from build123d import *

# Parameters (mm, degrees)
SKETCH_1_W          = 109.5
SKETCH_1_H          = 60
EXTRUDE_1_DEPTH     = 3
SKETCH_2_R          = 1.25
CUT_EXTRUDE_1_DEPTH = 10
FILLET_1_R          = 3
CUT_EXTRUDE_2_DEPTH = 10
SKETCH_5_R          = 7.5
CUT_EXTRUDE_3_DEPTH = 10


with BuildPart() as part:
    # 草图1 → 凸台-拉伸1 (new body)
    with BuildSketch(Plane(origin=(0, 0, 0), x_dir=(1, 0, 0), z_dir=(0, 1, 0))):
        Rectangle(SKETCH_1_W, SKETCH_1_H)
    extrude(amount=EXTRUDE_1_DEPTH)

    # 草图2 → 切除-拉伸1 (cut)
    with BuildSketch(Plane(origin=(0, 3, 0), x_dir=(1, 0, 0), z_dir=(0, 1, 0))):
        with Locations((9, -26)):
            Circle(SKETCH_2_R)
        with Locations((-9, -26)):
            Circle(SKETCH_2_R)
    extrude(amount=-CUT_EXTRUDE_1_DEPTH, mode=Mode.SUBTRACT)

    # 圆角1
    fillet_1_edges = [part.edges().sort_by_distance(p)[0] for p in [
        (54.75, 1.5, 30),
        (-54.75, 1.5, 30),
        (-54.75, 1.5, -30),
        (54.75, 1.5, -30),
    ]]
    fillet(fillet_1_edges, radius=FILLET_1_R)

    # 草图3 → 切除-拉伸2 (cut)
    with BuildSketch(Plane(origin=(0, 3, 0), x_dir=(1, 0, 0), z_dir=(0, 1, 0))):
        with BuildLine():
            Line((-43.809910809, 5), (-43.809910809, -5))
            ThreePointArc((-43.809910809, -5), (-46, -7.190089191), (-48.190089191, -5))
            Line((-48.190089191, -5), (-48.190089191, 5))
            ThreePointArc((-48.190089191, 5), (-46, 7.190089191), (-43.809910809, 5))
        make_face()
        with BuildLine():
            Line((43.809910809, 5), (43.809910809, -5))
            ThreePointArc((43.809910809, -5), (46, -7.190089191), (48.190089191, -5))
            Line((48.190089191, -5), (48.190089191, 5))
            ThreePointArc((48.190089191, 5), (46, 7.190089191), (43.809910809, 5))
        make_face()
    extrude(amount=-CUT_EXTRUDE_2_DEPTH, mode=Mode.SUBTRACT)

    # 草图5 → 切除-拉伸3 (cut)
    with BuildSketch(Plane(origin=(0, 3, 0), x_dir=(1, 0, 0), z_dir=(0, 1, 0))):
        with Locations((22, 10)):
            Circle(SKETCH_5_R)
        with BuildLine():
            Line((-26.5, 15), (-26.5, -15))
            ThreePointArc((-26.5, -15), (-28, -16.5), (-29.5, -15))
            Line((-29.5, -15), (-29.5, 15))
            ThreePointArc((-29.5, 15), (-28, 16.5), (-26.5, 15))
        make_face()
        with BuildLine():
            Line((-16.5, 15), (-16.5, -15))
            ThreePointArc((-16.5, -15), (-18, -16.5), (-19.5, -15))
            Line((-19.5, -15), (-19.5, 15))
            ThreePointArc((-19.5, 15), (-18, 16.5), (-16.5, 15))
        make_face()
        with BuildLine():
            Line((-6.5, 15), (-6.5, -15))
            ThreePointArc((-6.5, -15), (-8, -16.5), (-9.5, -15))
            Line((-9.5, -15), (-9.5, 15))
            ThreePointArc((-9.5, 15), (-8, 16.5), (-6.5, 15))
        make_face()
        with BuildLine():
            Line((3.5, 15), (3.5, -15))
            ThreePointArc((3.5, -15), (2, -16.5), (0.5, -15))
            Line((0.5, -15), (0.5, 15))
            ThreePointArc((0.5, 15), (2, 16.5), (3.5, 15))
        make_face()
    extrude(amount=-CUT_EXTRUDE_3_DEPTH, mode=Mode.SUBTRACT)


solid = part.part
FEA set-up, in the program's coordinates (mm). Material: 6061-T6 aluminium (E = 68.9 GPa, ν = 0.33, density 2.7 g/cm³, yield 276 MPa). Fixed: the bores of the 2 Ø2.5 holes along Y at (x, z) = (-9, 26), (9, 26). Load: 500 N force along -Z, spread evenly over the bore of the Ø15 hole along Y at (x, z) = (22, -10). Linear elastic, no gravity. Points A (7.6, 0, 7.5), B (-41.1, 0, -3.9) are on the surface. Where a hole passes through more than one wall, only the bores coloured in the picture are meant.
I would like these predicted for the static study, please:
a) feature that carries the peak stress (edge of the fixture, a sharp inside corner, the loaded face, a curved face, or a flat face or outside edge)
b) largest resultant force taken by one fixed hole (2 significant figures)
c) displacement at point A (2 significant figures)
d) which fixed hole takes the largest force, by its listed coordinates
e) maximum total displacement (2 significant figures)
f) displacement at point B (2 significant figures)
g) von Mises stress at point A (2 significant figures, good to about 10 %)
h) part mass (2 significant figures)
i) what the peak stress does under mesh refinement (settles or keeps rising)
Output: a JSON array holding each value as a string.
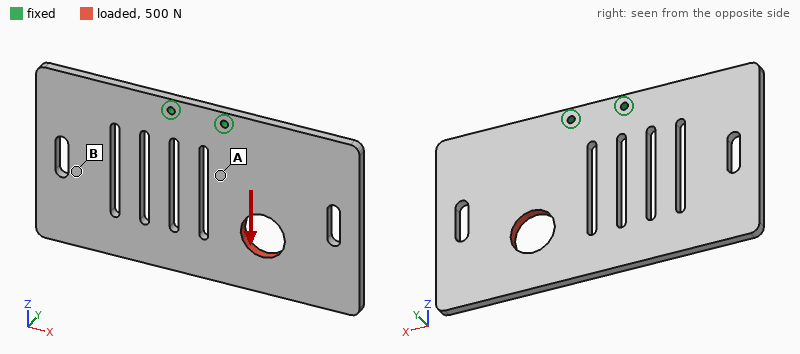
["edge of the fixture", "800 N", "11 µm", "(9, 26)", "48 µm", "26 µm", "8.1 MPa", "48 g", "keeps rising"]
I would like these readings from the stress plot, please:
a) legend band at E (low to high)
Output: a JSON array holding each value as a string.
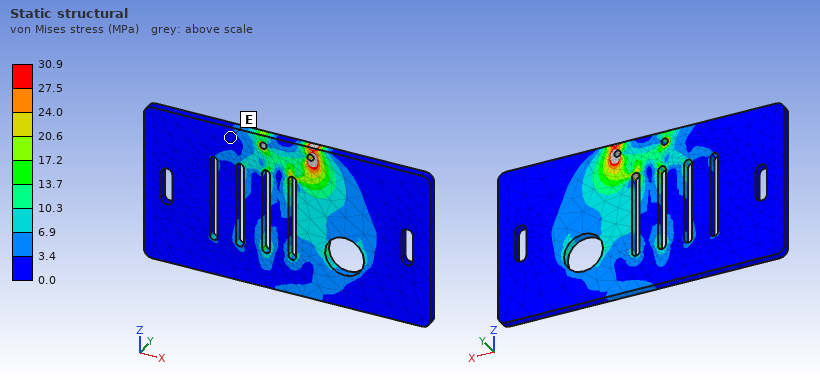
["0.0 to 3.4 MPa"]
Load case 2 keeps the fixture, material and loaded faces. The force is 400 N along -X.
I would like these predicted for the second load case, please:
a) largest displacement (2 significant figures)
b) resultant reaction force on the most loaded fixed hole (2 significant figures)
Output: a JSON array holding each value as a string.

["81 µm", "750 N"]
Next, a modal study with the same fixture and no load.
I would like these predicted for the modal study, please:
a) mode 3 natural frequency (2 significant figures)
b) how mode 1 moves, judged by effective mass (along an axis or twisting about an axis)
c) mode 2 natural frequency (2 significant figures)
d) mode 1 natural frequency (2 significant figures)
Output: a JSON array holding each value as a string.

["1000 Hz", "along Y", "550 Hz", "480 Hz"]
